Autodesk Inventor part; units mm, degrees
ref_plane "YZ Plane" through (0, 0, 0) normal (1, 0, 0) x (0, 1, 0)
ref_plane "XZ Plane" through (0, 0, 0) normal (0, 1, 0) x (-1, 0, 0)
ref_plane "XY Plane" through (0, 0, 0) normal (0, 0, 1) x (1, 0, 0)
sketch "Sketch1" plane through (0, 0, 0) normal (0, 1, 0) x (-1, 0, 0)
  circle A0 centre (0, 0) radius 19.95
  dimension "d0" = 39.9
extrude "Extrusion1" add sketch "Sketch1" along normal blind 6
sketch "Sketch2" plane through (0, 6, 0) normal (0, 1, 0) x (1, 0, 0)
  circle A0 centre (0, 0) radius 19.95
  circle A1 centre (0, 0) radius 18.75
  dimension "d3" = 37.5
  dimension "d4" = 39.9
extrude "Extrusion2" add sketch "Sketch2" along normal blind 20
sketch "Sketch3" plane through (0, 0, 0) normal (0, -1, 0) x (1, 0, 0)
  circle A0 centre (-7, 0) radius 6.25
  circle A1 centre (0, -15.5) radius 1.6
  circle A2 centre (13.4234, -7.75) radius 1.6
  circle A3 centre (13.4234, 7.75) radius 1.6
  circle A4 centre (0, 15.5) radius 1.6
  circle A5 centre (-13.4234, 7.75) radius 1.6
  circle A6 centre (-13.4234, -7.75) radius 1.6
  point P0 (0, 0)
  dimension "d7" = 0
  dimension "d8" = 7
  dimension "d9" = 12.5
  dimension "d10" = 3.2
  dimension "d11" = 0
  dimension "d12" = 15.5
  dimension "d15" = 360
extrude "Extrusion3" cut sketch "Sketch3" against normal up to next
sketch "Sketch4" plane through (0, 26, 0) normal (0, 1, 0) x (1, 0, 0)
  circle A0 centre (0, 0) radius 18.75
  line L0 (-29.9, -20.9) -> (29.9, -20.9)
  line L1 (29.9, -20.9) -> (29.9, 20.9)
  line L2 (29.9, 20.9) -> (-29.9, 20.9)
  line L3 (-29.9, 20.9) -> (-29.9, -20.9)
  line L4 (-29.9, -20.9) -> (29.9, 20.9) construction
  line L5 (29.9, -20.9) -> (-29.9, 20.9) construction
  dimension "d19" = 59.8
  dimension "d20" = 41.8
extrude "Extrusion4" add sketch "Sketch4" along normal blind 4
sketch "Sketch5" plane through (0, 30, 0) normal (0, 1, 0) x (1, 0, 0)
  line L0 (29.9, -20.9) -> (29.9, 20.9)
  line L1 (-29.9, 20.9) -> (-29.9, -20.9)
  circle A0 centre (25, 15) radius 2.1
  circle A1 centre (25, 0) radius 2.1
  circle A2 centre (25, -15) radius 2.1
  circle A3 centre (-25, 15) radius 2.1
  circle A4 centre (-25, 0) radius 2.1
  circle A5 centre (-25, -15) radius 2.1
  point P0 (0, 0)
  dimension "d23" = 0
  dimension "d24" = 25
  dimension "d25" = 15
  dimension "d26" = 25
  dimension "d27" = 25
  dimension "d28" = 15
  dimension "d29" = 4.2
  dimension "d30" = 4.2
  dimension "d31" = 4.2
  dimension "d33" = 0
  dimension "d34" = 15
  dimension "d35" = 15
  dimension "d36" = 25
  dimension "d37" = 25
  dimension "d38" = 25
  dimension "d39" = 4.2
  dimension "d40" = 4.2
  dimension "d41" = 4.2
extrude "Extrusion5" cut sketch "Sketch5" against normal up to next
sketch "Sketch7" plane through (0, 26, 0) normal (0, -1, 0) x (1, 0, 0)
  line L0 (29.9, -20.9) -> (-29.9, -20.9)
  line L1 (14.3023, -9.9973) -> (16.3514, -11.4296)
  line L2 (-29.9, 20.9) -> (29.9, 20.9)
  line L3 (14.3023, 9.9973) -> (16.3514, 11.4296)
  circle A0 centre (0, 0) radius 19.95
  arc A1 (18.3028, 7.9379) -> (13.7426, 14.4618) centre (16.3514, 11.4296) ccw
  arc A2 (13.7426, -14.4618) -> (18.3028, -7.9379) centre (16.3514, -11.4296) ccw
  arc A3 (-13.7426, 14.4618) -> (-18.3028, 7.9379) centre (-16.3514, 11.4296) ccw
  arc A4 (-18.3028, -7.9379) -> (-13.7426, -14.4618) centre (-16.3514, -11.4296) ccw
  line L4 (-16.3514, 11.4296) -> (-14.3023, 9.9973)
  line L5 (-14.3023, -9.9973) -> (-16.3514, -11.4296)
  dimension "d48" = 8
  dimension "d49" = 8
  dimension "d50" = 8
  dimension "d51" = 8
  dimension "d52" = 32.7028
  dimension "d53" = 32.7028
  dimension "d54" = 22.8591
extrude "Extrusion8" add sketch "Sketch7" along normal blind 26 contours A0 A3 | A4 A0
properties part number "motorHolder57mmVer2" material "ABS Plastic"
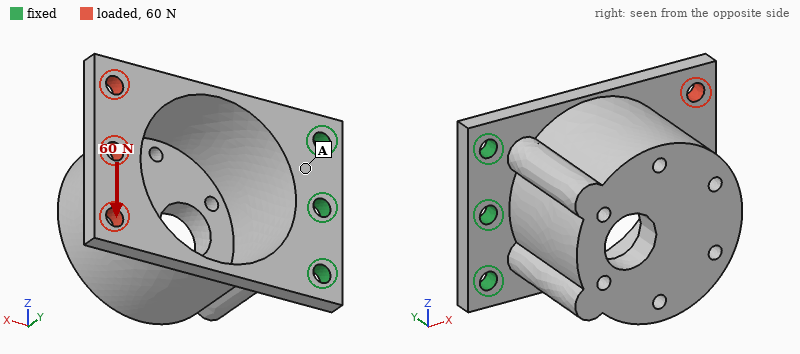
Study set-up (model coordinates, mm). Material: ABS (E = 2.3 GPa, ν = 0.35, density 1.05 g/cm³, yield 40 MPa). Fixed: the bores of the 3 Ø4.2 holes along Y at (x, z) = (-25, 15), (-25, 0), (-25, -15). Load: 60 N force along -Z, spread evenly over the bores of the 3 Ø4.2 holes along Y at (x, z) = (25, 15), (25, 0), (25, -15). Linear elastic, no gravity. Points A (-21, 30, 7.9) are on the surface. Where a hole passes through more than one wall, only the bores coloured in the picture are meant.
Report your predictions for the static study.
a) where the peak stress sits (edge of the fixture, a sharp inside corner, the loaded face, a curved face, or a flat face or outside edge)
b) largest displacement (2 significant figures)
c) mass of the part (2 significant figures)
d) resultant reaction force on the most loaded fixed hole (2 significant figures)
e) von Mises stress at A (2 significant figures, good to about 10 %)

a flat face or outside edge
0.91 mm
17 g
85 N
3.5 MPa
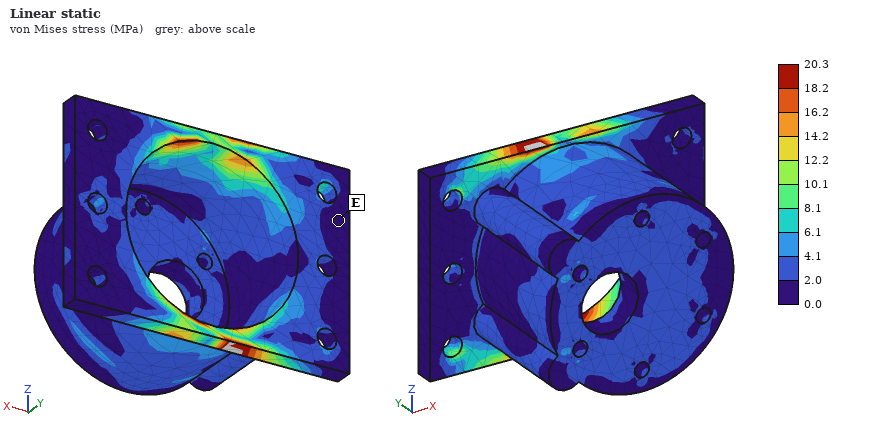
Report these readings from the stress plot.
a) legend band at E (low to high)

0.0 to 2.0 MPa
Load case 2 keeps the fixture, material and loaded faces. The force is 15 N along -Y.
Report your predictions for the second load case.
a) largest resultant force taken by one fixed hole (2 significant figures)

12 N
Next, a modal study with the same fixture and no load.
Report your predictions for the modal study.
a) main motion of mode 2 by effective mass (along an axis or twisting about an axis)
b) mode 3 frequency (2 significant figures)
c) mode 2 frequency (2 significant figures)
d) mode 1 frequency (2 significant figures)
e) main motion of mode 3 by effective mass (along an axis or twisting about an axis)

along Z
1300 Hz
620 Hz
270 Hz
along Z
